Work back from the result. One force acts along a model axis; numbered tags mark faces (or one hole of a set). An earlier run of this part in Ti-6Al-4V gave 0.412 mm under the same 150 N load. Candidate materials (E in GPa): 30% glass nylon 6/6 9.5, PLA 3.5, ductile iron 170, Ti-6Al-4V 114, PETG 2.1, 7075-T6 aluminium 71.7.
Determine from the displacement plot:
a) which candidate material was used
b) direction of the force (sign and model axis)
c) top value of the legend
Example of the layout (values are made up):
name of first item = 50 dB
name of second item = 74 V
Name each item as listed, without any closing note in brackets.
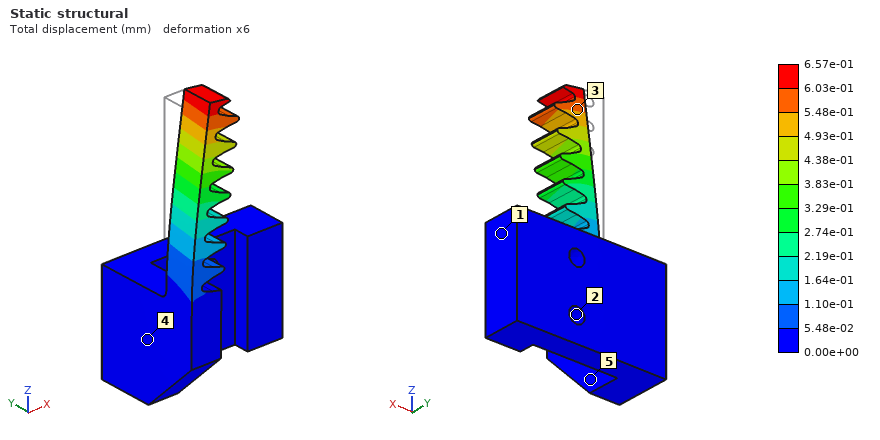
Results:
which candidate material was used = 7075-T6 aluminium
direction of the force = +X
top value of the legend = 6.57e-01 mm
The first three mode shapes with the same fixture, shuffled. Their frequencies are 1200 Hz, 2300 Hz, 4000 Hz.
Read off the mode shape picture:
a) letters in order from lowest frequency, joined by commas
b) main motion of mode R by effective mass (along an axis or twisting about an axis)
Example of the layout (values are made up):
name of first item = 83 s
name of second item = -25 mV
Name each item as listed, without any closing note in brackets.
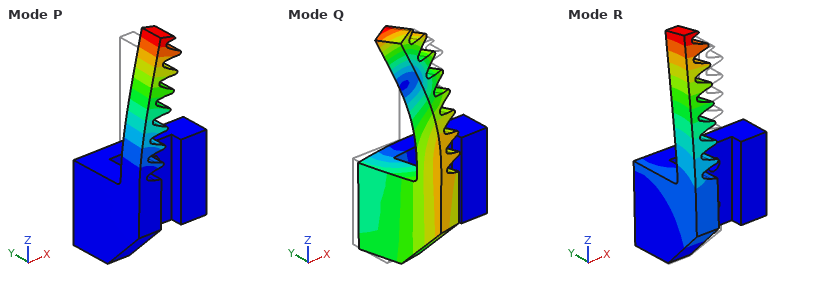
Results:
letters in order from lowest frequency, joined by commas = P, R, Q
main motion of mode R by effective mass = along Y
